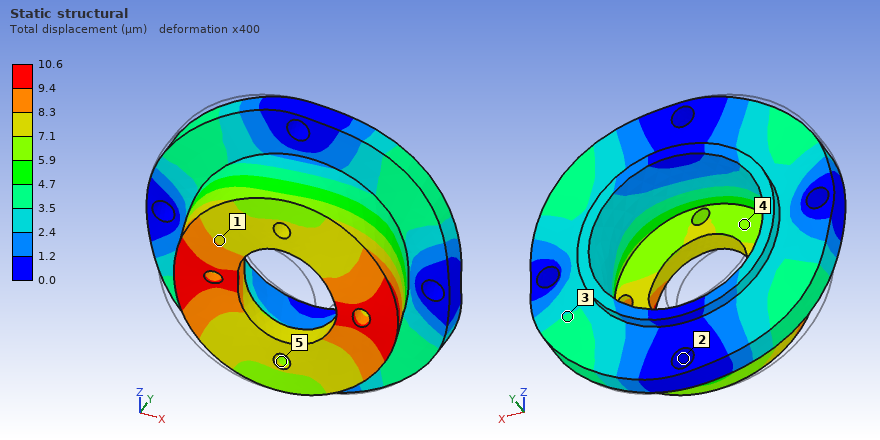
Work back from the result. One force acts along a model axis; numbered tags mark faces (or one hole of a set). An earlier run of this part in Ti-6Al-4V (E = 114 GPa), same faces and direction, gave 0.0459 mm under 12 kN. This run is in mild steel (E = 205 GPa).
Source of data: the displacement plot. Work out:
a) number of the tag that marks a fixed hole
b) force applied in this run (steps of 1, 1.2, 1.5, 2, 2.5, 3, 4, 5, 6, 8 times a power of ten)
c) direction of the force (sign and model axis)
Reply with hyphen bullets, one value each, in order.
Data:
- 2
- 5 kN
- +X
